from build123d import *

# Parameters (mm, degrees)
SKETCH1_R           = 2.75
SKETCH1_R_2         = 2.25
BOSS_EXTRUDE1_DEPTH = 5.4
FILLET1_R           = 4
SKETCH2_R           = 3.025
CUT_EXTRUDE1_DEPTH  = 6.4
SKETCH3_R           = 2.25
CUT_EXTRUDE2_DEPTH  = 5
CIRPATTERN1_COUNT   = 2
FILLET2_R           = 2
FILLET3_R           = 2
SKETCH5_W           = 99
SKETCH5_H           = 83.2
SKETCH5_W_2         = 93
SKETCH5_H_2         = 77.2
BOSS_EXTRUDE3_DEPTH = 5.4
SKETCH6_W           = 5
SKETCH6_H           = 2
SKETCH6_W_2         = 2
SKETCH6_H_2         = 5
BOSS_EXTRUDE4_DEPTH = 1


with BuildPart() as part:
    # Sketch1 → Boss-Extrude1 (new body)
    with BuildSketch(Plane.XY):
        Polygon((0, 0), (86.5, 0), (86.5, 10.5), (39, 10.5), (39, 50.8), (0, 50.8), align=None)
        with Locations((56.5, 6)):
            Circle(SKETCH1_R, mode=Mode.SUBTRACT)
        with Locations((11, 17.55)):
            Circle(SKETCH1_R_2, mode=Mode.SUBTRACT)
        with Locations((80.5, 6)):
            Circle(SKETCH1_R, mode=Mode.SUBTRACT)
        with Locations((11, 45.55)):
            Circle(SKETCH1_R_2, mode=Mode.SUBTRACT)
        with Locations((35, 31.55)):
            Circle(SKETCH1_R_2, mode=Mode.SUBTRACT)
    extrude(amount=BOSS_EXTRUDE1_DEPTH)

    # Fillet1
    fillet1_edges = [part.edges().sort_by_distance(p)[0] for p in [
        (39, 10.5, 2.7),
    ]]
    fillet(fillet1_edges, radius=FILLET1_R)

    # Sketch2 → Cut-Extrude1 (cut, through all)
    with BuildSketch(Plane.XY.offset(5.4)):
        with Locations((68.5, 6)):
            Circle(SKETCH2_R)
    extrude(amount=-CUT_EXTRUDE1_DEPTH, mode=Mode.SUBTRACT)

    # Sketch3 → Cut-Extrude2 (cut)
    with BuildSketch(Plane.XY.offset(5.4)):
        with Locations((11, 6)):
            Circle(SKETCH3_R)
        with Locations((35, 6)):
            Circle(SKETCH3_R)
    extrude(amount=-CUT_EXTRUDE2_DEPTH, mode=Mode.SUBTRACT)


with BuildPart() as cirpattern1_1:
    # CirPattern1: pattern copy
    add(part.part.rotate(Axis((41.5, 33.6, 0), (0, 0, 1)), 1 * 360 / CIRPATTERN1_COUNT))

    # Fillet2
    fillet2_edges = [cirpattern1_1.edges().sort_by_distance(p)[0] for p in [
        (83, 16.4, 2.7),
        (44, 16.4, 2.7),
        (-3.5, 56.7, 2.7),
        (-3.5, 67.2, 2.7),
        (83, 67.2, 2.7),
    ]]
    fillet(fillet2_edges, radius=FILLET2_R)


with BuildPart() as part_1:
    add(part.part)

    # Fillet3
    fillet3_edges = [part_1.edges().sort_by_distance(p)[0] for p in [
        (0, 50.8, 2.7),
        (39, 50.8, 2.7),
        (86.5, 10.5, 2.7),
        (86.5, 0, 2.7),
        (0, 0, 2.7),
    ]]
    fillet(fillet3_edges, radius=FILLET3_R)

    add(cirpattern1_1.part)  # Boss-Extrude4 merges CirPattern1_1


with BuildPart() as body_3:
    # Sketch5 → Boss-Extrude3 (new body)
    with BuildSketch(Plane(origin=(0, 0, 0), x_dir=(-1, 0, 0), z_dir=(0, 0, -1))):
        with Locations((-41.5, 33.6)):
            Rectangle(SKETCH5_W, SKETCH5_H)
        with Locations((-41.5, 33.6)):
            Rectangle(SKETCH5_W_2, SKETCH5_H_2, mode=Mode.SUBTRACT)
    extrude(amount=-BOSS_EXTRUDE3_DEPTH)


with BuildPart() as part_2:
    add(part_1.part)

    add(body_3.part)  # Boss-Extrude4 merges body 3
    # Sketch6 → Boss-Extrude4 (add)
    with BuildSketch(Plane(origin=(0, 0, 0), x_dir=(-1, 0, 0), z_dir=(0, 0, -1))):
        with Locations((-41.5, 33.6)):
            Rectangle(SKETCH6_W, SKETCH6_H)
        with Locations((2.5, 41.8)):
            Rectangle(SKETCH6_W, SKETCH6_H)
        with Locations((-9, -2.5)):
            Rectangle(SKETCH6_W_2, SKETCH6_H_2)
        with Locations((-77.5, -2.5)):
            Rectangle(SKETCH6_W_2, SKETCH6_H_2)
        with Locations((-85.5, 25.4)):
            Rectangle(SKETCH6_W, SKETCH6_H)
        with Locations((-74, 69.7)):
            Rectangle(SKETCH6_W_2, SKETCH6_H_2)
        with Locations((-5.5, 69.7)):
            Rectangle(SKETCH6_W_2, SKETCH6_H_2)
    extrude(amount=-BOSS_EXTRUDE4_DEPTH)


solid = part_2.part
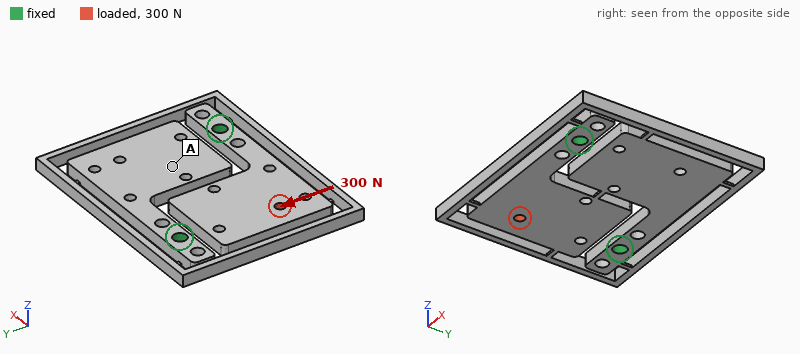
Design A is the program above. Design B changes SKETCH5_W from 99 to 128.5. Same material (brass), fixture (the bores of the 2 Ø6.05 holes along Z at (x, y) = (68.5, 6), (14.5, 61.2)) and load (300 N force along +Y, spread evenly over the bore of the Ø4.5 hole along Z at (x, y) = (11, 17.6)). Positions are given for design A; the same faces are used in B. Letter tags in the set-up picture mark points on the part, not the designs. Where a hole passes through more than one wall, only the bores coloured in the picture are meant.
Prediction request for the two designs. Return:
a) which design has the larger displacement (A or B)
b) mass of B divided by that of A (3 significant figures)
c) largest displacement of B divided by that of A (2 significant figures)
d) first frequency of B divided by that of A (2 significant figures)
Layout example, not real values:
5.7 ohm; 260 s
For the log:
A; 1.43; 0.66; 0.63
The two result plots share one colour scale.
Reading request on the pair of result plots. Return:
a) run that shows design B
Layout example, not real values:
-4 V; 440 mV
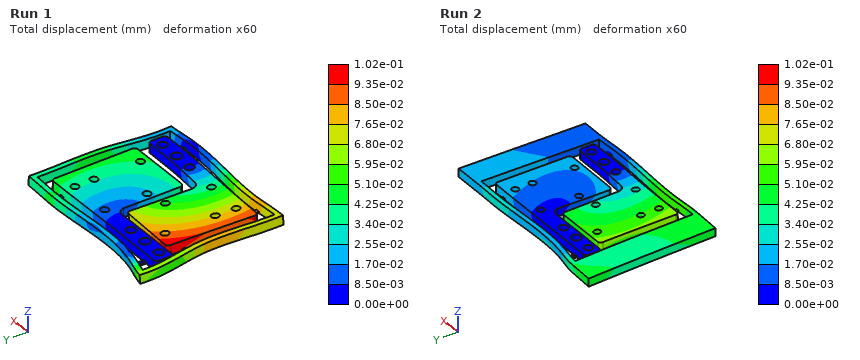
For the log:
Run 2
